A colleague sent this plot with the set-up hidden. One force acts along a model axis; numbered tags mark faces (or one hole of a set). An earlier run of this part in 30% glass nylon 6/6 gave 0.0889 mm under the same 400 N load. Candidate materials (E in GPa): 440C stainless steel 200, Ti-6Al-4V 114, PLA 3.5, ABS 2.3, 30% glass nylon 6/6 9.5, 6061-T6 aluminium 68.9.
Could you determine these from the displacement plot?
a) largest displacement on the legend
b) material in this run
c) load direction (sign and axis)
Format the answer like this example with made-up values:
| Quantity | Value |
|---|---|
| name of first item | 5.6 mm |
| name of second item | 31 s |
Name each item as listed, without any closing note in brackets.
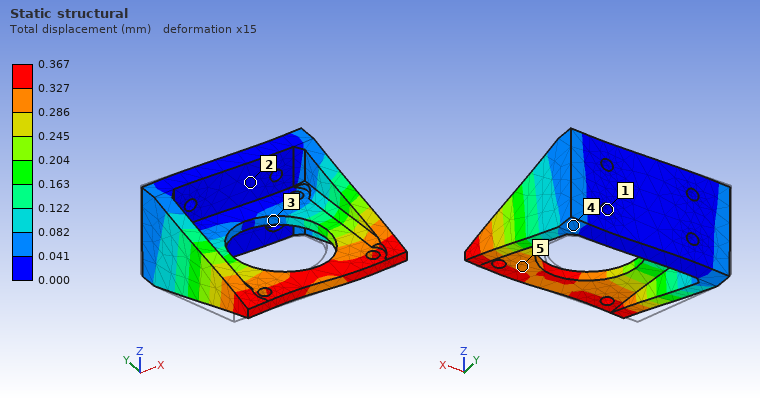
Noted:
| Quantity | Value |
|---|---|
| largest displacement on the legend | 0.367 mm |
| material in this run | ABS |
| load direction | +X |
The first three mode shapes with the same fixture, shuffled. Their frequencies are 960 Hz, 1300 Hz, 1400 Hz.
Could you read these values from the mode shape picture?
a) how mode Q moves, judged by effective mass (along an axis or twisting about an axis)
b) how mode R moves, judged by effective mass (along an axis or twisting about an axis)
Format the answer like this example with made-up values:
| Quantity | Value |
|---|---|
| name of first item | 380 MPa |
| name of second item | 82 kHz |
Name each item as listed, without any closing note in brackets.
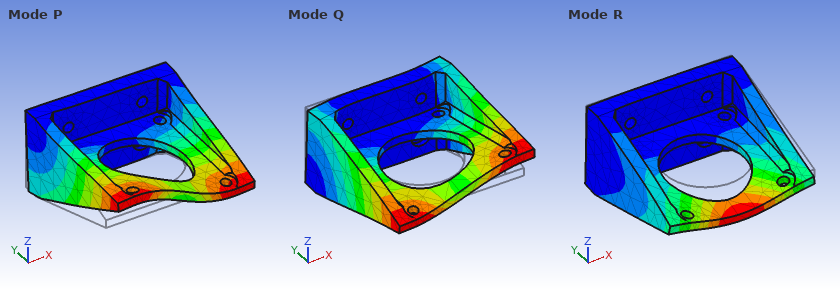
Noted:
| Quantity | Value |
|---|---|
| how mode Q moves, judged by effective mass | along X |
| how mode R moves, judged by effective mass | along Z |
